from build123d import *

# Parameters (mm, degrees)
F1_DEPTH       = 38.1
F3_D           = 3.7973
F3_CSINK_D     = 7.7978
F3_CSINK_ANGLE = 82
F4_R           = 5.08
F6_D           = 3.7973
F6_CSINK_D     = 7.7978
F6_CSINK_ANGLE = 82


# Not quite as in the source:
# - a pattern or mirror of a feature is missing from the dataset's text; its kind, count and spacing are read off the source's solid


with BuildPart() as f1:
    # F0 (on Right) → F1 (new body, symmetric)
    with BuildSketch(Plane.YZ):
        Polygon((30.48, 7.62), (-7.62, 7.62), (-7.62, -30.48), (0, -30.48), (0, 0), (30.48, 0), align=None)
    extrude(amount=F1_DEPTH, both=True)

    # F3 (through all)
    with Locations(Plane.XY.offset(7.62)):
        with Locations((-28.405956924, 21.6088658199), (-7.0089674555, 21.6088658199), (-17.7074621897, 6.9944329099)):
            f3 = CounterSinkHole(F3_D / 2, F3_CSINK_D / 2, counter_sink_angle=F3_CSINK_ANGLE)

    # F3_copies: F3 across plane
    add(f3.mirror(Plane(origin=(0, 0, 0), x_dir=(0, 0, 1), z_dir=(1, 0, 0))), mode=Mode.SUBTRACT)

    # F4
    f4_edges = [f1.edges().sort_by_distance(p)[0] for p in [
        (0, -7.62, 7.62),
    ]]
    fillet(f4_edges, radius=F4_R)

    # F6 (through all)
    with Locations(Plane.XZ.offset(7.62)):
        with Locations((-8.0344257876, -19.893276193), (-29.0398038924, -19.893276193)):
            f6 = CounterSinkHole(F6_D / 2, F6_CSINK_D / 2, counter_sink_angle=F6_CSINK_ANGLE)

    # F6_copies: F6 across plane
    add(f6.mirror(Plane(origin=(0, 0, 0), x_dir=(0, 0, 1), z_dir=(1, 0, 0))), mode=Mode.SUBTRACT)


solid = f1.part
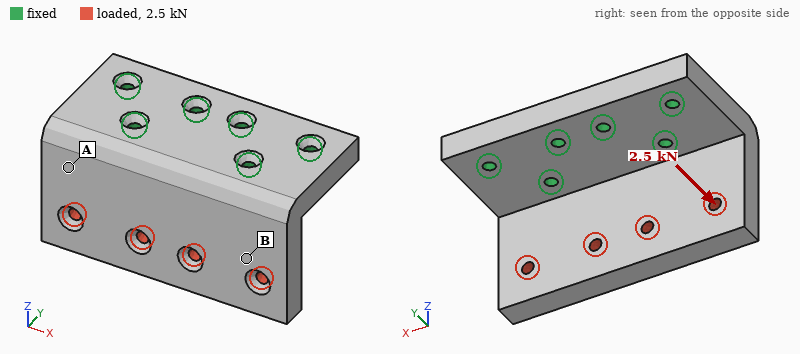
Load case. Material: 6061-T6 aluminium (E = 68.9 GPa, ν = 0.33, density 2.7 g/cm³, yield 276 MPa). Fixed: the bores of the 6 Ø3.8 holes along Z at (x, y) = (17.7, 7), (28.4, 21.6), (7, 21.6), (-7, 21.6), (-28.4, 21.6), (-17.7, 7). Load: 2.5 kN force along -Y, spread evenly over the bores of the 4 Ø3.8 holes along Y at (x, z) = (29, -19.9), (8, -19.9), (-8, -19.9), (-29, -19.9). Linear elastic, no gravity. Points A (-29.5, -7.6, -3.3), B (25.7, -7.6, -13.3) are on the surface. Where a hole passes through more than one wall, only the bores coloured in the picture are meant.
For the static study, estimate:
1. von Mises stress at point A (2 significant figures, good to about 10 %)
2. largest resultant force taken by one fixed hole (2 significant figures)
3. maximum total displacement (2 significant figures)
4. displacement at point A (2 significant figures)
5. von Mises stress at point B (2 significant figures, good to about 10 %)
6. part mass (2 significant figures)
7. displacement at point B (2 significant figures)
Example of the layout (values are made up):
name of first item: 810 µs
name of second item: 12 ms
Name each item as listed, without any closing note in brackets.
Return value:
von Mises stress at point A: 48 MPa
largest resultant force taken by one fixed hole: 1.7 kN
maximum total displacement: 0.22 mm
displacement at point A: 0.062 mm
von Mises stress at point B: 21 MPa
part mass: 100 g
displacement at point B: 0.11 mm
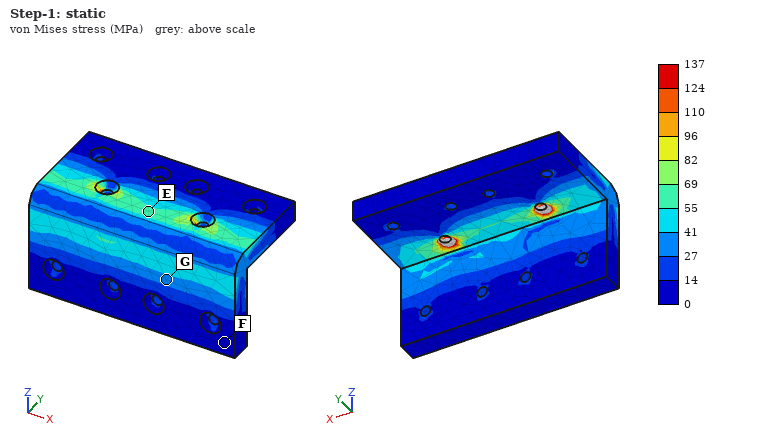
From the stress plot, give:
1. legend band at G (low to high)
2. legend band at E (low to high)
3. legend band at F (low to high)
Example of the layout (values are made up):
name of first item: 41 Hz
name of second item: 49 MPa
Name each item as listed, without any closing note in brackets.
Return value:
legend band at G: 27 to 41 MPa
legend band at E: 55 to 69 MPa
legend band at F: 0 to 14 MPa
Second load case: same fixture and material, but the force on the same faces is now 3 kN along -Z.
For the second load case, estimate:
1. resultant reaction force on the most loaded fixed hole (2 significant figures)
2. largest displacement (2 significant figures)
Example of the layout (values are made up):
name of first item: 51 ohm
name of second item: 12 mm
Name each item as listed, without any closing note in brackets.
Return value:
resultant reaction force on the most loaded fixed hole: 1.9 kN
largest displacement: 50 µm
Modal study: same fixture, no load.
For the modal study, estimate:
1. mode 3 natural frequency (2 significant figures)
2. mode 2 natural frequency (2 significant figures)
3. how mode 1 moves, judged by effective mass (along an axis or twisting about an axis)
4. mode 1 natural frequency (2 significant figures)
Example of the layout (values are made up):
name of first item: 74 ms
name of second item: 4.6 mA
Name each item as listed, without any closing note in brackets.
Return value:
mode 3 natural frequency: 7900 Hz
mode 2 natural frequency: 5100 Hz
how mode 1 moves, judged by effective mass: along Y
mode 1 natural frequency: 3300 Hz
